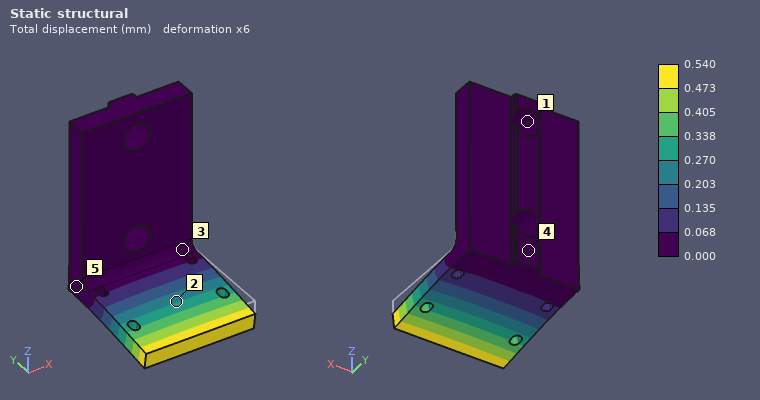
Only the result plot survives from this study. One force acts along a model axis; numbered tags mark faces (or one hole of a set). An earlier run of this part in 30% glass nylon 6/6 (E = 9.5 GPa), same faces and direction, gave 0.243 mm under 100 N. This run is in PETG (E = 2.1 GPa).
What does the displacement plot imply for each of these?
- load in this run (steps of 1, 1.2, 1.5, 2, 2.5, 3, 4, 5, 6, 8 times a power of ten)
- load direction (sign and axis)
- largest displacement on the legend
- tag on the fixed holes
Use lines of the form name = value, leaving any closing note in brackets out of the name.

load in this run = 50 N
load direction = -Z
largest displacement on the legend = 0.540 mm
tag on the fixed holes = 1
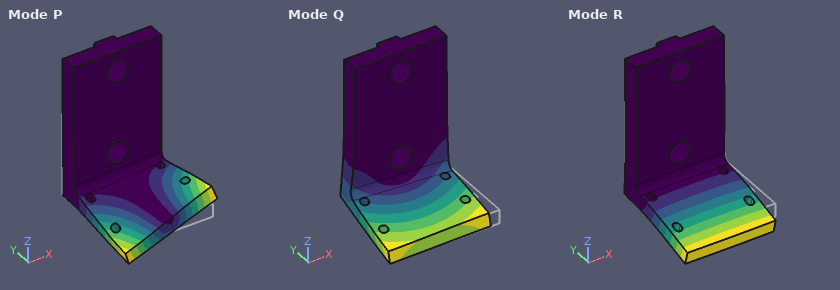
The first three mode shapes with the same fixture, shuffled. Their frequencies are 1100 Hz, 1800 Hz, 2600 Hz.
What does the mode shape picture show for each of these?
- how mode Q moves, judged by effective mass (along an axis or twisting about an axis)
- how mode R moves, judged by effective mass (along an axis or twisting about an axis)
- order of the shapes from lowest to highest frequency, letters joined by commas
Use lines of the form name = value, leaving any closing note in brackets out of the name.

how mode Q moves, judged by effective mass = along X
how mode R moves, judged by effective mass = along Z
order of the shapes from lowest to highest frequency, letters joined by commas = R, Q, P
